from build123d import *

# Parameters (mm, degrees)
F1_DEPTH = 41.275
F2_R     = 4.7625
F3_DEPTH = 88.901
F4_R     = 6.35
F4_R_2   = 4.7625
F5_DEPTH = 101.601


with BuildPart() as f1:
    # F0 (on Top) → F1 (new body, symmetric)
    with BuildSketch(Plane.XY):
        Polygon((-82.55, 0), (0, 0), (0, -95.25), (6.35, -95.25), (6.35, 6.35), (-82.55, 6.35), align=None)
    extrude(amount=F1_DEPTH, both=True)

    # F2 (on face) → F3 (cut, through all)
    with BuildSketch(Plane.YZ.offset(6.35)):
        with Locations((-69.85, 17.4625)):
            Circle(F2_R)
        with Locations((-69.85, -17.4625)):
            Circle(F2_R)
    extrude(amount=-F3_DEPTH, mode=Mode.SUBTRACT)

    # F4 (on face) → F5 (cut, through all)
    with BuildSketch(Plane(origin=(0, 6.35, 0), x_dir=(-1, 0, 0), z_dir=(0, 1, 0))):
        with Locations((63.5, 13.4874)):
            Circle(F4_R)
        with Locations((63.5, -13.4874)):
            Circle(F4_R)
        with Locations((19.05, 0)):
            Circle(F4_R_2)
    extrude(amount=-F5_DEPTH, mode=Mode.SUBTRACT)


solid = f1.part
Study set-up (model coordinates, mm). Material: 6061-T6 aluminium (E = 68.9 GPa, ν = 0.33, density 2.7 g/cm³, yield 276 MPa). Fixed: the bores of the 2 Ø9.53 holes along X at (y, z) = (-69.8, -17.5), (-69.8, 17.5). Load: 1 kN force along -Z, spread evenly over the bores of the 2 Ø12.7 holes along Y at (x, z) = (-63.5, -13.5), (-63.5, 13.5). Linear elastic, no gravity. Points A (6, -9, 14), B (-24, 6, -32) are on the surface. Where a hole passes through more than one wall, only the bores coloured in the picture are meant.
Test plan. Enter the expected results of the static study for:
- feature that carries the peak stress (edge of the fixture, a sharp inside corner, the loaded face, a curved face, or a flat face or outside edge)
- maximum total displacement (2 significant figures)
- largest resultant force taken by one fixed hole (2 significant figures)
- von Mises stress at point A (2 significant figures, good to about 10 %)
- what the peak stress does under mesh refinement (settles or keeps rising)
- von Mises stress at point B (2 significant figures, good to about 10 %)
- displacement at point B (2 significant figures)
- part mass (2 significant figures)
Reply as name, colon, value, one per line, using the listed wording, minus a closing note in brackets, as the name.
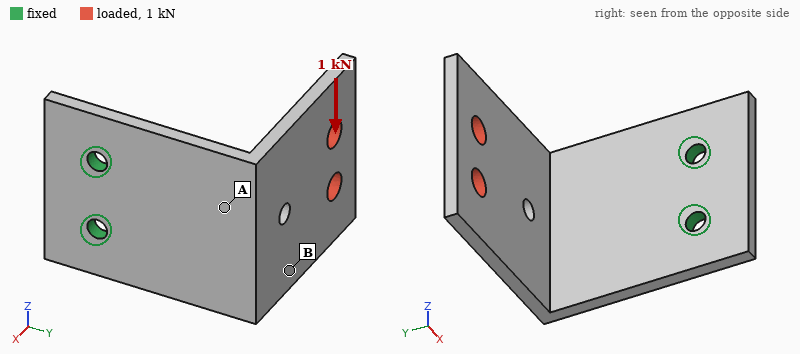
feature that carries the peak stress: edge of the fixture
maximum total displacement: 1.7 mm
largest resultant force taken by one fixed hole: 2.2 kN
von Mises stress at point A: 69 MPa
what the peak stress does under mesh refinement: keeps rising
von Mises stress at point B: 18 MPa
displacement at point B: 0.75 mm
part mass: 250 g
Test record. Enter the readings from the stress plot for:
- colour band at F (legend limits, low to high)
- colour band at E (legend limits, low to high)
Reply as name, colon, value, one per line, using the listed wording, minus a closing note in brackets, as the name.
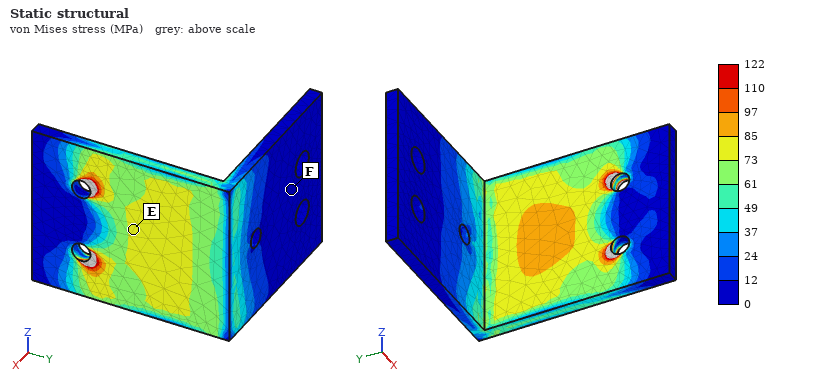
colour band at F: 0 to 12 MPa
colour band at E: 73 to 85 MPa
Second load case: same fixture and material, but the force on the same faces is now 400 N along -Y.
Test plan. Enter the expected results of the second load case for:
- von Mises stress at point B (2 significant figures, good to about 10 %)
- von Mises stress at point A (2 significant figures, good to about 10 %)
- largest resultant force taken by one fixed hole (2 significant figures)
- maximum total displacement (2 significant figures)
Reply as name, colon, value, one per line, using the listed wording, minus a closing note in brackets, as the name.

von Mises stress at point B: 30 MPa
von Mises stress at point A: 43 MPa
largest resultant force taken by one fixed hole: 200 N
maximum total displacement: 1.8 mm
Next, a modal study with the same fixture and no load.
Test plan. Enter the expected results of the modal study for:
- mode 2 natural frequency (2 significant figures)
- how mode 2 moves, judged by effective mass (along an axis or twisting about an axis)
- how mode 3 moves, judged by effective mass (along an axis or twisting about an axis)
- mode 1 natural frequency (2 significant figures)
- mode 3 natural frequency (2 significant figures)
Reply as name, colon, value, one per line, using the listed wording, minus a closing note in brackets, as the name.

mode 2 natural frequency: 510 Hz
how mode 2 moves, judged by effective mass: along Z
how mode 3 moves, judged by effective mass: along X
mode 1 natural frequency: 290 Hz
mode 3 natural frequency: 800 Hz
